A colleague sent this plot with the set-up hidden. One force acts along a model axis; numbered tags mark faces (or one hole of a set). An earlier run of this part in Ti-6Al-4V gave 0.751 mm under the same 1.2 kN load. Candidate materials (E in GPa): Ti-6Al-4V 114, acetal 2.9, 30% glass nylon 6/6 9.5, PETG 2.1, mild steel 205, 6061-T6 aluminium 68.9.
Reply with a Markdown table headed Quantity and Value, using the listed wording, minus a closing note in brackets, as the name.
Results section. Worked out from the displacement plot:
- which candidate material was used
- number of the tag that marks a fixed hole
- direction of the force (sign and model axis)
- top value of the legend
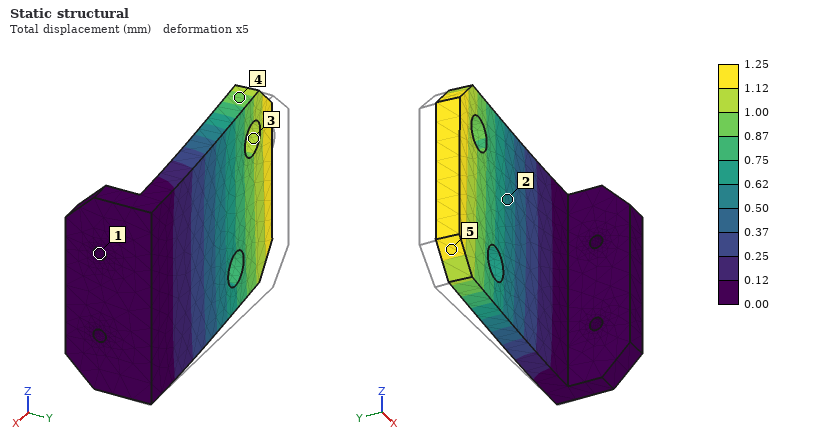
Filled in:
| Quantity | Value |
|---|---|
| which candidate material was used | 6061-T6 aluminium |
| number of the tag that marks a fixed hole | 1 |
| direction of the force | -Y |
| top value of the legend | 1.25 mm |
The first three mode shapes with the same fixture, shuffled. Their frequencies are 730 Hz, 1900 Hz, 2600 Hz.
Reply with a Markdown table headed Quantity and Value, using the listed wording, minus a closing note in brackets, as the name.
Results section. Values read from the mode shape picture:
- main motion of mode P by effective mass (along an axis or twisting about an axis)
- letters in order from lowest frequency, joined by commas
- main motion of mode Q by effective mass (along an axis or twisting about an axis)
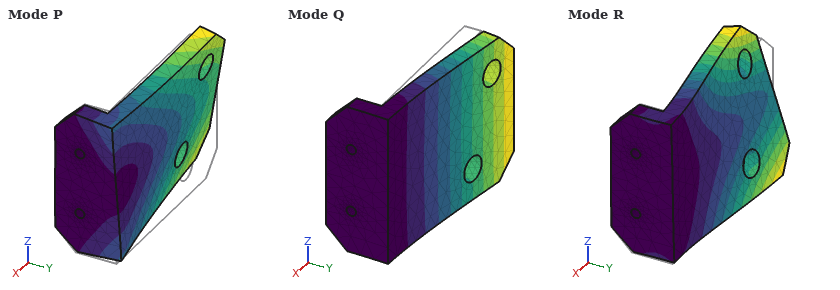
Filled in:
| Quantity | Value |
|---|---|
| main motion of mode P by effective mass | along Z |
| letters in order from lowest frequency, joined by commas | Q, P, R |
| main motion of mode Q by effective mass | along Y |
